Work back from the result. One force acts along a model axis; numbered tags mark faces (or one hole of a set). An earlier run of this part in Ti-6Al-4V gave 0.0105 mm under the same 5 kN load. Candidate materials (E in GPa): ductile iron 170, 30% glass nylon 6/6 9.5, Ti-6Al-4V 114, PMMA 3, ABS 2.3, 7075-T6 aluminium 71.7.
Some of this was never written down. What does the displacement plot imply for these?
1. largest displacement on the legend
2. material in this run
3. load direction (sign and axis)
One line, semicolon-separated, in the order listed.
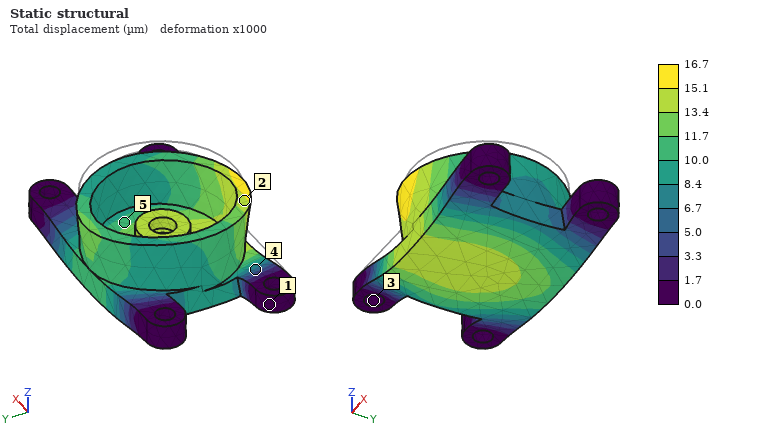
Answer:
16.7 µm; 7075-T6 aluminium; -Z
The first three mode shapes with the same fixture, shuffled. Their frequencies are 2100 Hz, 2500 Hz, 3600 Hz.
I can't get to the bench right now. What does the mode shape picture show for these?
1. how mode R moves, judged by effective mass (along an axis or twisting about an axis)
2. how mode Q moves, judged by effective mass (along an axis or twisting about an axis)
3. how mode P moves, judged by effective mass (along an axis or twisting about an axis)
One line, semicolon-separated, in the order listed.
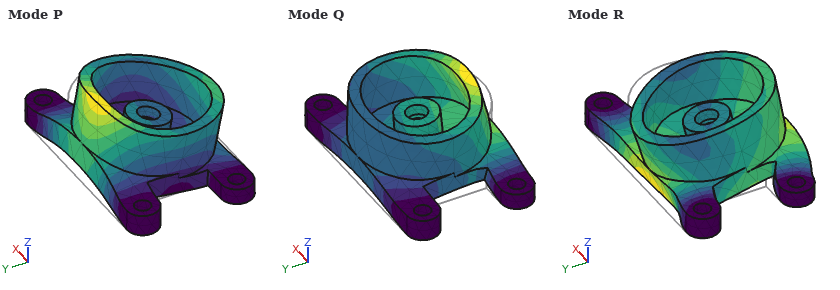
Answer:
along Y; along Z; along Y
